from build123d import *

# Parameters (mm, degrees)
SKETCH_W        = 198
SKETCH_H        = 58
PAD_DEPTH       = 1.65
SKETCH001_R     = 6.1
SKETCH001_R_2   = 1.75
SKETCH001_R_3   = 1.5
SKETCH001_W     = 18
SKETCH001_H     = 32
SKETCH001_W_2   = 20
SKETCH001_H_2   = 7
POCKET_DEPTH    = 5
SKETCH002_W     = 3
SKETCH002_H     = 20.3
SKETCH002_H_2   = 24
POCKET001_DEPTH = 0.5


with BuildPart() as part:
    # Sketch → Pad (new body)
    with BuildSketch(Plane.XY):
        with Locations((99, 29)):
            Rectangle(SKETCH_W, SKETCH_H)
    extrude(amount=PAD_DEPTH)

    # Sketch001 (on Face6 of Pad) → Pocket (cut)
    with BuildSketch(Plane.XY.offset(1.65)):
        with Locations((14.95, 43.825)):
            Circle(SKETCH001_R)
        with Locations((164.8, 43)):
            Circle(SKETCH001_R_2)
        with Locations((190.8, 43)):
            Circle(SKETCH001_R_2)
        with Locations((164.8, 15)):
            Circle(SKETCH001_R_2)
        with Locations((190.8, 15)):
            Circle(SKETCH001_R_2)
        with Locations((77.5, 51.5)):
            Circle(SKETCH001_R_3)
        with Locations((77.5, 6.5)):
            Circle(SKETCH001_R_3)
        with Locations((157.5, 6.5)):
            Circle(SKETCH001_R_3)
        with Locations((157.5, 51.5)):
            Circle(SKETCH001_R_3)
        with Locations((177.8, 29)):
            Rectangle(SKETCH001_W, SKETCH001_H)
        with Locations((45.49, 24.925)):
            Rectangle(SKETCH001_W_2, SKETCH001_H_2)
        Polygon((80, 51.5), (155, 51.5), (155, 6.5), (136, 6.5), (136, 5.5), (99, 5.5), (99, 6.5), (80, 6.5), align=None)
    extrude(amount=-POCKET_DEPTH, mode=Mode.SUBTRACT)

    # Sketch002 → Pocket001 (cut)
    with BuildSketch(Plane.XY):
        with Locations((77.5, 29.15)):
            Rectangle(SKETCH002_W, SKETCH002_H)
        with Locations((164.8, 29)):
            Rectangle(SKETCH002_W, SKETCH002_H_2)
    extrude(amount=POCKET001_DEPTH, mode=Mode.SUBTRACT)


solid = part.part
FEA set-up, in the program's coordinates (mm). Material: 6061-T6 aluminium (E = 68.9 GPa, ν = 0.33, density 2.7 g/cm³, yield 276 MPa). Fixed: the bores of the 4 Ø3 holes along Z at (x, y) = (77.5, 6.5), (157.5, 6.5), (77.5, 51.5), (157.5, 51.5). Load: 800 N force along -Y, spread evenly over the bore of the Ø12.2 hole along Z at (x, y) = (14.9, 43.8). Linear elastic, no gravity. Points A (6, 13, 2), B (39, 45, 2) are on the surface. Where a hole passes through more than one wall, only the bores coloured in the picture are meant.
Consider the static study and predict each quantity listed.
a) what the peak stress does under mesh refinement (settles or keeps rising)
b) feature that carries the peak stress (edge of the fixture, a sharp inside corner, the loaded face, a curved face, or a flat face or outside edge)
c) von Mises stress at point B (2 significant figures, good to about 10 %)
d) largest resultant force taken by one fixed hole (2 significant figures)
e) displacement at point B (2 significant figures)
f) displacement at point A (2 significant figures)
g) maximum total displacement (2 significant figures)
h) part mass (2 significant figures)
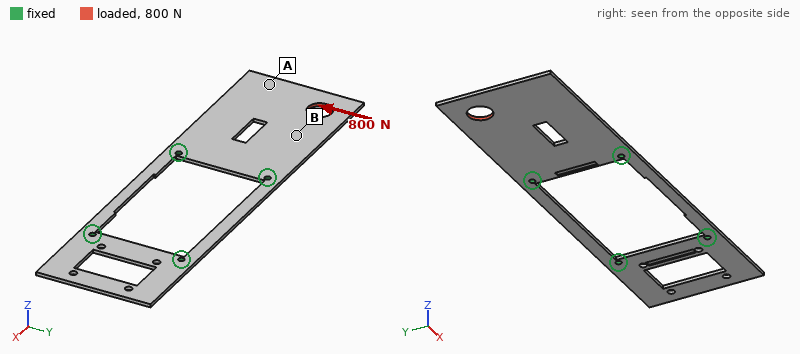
keeps rising
edge of the fixture
23 MPa
1.1 kN
0.047 mm
0.088 mm
0.10 mm
32 g
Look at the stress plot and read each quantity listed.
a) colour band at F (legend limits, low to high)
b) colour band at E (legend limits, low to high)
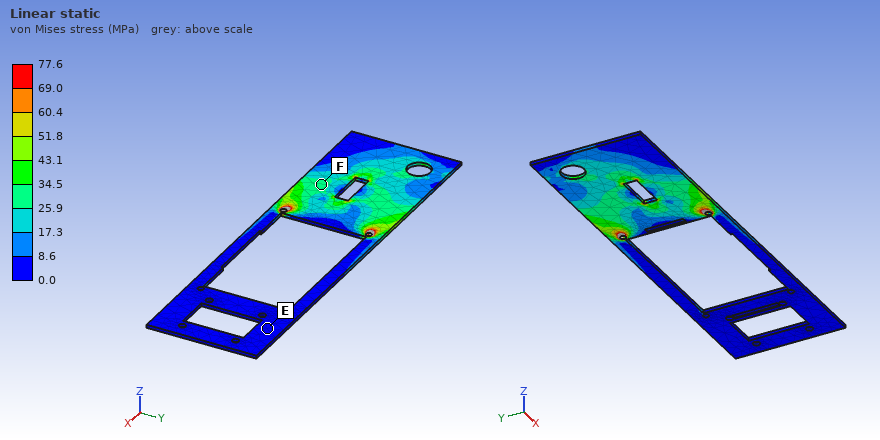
25.9 to 34.5 MPa
0.0 to 8.6 MPa
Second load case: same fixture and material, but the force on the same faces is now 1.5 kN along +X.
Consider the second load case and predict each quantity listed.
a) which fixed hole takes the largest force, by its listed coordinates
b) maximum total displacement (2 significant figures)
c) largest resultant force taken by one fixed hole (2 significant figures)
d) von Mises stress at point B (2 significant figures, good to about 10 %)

(77.5, 51.5)
55 µm
1.2 kN
30 MPa
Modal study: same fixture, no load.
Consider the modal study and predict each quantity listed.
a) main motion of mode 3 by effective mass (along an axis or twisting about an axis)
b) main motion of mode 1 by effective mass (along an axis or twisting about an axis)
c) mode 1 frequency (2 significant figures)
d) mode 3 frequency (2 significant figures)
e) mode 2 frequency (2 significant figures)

twisting about X
along Z
200 Hz
690 Hz
640 Hz
